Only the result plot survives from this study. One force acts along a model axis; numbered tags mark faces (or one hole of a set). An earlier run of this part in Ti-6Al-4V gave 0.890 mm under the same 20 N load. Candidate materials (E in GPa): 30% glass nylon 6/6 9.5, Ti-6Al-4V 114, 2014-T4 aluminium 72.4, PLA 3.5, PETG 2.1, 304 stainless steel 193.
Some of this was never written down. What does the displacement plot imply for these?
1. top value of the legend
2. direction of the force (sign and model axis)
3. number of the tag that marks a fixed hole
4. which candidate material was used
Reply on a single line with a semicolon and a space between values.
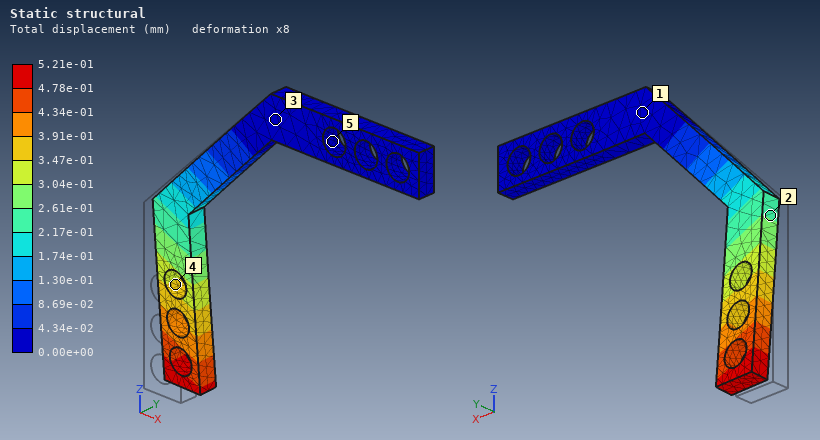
5.21e-01 mm; +Y; 5; 304 stainless steel
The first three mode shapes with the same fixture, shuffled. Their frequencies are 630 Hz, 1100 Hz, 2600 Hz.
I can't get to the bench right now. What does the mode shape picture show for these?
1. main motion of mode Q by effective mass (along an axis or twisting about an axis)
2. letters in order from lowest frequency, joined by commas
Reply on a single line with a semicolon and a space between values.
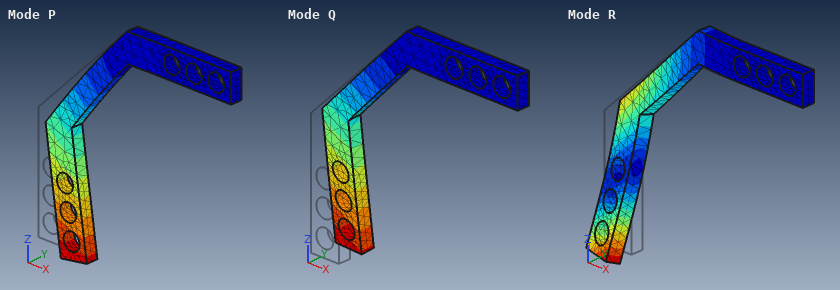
along Y; Q, P, R
